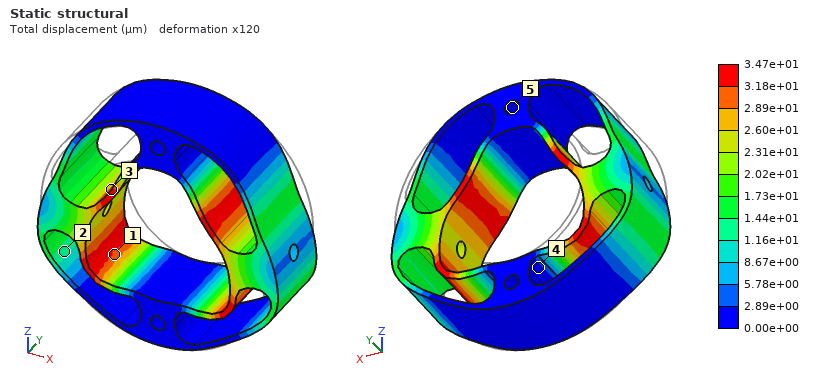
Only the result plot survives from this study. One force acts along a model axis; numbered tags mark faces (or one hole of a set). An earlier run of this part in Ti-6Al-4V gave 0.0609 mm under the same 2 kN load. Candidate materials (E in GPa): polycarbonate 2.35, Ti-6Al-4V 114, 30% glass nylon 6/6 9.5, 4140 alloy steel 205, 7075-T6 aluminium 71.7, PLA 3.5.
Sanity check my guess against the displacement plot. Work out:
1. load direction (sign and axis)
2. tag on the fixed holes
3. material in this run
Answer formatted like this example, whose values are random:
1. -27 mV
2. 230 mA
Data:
1. -Z
2. 5
3. 4140 alloy steel
